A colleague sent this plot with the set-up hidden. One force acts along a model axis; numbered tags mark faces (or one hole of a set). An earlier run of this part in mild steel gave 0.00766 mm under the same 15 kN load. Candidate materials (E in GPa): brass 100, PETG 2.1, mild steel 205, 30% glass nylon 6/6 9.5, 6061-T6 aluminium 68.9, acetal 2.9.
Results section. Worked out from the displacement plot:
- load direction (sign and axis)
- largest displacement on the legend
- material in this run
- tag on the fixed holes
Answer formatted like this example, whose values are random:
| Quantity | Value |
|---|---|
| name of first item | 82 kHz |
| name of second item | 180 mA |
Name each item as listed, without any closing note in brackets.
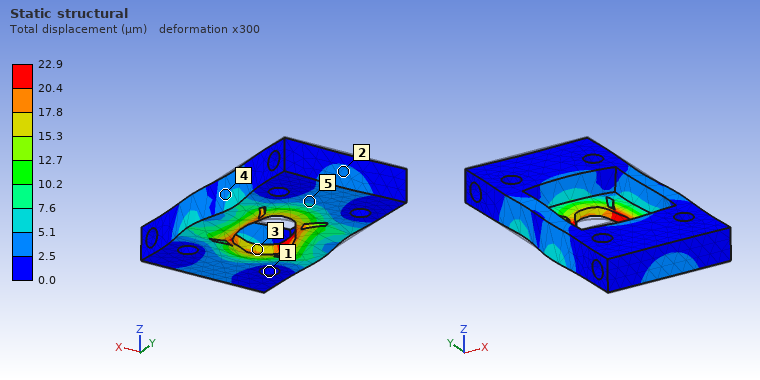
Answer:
| Quantity | Value |
|---|---|
| load direction | -Y |
| largest displacement on the legend | 22.9 µm |
| material in this run | 6061-T6 aluminium |
| tag on the fixed holes | 1 |
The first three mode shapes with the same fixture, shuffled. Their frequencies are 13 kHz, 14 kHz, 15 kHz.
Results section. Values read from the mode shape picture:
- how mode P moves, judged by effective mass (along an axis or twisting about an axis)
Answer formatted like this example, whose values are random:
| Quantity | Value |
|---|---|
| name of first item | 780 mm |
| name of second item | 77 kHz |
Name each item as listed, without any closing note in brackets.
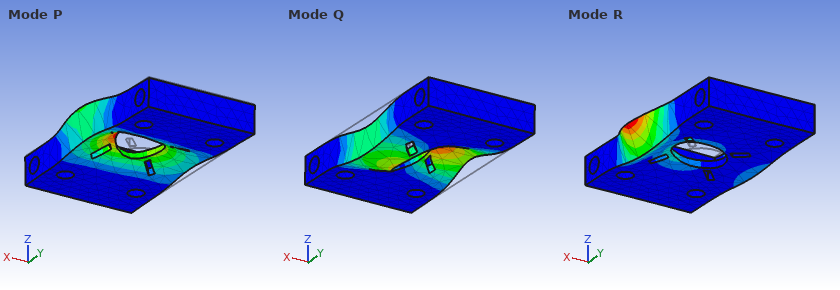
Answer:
| Quantity | Value |
|---|---|
| how mode P moves, judged by effective mass | along Z |
